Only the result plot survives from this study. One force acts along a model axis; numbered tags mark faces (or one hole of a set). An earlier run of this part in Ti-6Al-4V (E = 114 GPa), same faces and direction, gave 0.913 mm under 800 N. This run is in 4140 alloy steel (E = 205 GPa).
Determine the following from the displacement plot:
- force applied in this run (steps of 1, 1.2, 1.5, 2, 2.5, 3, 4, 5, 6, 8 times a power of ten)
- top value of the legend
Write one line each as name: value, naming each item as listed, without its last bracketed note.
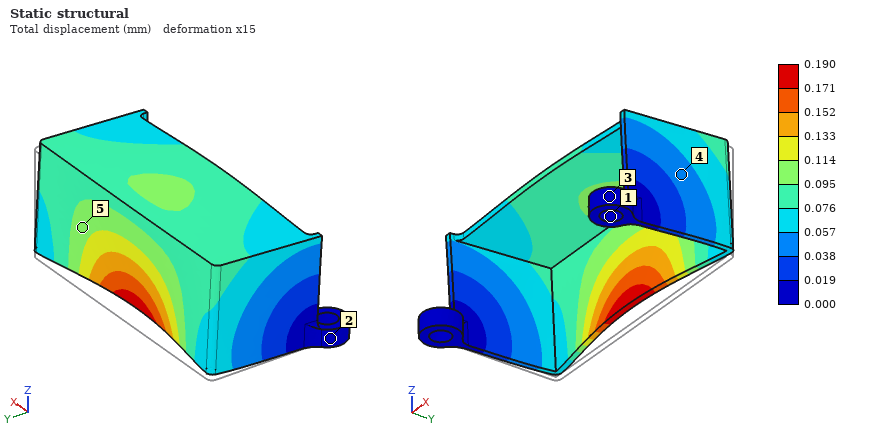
force applied in this run: 300 N
top value of the legend: 0.190 mm
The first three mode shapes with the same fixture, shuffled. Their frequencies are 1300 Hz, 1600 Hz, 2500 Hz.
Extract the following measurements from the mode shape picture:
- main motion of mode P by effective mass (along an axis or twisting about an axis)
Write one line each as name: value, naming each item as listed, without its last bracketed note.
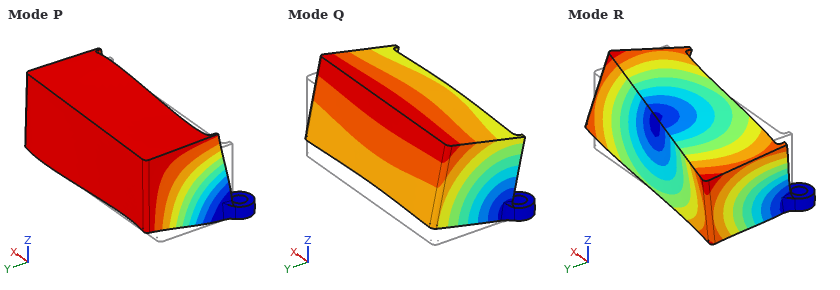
main motion of mode P by effective mass: along X
